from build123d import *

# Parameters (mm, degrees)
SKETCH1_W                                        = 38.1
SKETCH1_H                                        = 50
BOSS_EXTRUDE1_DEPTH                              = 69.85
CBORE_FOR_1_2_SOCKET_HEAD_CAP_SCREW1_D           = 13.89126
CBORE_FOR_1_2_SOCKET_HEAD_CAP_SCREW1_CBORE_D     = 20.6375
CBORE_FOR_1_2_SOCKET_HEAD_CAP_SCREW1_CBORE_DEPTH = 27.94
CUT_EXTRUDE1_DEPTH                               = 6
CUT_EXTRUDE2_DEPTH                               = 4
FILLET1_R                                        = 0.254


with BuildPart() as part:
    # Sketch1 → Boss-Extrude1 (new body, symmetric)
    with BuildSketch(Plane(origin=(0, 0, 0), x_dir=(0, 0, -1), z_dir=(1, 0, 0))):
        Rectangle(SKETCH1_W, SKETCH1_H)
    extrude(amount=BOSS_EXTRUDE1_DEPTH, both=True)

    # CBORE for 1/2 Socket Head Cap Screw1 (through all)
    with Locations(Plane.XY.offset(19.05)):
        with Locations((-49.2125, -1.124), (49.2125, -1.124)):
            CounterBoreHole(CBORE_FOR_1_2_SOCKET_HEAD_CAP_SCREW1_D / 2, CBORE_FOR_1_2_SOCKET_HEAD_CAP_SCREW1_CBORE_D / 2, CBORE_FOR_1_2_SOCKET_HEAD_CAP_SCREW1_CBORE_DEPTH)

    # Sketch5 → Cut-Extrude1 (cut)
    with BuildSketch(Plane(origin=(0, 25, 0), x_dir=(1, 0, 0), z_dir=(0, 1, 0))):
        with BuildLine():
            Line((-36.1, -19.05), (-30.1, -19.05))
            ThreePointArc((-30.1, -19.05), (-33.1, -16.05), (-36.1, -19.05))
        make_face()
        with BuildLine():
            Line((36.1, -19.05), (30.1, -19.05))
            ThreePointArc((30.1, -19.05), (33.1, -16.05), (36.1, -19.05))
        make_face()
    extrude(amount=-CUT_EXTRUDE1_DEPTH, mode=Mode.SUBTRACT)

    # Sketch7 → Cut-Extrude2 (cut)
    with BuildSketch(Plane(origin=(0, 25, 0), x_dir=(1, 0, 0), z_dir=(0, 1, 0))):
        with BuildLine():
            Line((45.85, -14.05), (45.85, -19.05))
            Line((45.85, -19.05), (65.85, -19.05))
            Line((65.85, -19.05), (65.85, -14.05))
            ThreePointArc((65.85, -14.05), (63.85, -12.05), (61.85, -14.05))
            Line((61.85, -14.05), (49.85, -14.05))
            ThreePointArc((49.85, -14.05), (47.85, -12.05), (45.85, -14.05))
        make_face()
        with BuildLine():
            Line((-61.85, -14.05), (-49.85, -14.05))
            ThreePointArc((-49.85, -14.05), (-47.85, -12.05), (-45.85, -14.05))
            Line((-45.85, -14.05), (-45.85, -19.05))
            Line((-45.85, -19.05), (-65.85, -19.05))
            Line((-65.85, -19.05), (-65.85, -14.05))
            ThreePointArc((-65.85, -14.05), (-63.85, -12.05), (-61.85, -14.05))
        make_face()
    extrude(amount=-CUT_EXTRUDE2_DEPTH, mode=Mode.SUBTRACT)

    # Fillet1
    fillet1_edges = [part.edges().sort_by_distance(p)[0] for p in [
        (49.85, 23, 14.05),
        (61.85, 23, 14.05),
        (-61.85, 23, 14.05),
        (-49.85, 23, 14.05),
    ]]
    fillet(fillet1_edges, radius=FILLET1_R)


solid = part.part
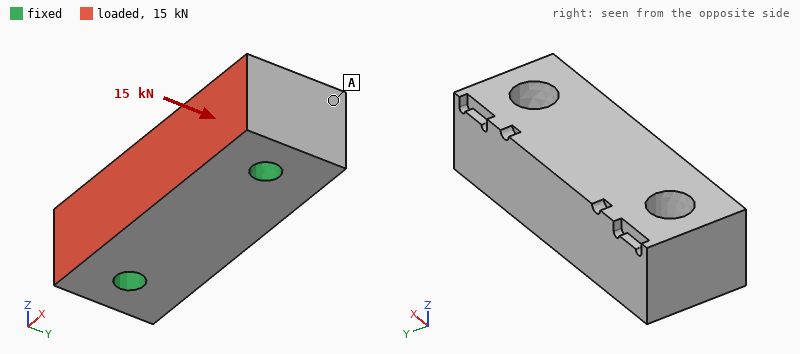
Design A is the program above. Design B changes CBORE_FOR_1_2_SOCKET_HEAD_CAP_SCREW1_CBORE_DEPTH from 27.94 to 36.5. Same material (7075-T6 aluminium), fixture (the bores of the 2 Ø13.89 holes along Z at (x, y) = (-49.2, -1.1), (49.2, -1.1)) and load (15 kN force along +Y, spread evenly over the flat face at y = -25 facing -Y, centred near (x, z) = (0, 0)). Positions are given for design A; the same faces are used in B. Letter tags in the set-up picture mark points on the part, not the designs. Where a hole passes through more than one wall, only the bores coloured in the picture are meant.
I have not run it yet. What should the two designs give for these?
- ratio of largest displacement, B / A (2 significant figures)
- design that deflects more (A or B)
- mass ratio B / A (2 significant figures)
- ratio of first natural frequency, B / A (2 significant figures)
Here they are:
17
B
0.99
0.25
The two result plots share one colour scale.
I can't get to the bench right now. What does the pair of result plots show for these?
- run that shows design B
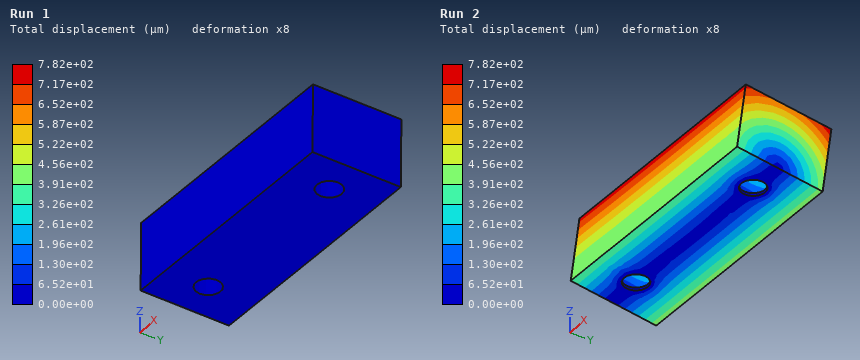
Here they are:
Run 2
